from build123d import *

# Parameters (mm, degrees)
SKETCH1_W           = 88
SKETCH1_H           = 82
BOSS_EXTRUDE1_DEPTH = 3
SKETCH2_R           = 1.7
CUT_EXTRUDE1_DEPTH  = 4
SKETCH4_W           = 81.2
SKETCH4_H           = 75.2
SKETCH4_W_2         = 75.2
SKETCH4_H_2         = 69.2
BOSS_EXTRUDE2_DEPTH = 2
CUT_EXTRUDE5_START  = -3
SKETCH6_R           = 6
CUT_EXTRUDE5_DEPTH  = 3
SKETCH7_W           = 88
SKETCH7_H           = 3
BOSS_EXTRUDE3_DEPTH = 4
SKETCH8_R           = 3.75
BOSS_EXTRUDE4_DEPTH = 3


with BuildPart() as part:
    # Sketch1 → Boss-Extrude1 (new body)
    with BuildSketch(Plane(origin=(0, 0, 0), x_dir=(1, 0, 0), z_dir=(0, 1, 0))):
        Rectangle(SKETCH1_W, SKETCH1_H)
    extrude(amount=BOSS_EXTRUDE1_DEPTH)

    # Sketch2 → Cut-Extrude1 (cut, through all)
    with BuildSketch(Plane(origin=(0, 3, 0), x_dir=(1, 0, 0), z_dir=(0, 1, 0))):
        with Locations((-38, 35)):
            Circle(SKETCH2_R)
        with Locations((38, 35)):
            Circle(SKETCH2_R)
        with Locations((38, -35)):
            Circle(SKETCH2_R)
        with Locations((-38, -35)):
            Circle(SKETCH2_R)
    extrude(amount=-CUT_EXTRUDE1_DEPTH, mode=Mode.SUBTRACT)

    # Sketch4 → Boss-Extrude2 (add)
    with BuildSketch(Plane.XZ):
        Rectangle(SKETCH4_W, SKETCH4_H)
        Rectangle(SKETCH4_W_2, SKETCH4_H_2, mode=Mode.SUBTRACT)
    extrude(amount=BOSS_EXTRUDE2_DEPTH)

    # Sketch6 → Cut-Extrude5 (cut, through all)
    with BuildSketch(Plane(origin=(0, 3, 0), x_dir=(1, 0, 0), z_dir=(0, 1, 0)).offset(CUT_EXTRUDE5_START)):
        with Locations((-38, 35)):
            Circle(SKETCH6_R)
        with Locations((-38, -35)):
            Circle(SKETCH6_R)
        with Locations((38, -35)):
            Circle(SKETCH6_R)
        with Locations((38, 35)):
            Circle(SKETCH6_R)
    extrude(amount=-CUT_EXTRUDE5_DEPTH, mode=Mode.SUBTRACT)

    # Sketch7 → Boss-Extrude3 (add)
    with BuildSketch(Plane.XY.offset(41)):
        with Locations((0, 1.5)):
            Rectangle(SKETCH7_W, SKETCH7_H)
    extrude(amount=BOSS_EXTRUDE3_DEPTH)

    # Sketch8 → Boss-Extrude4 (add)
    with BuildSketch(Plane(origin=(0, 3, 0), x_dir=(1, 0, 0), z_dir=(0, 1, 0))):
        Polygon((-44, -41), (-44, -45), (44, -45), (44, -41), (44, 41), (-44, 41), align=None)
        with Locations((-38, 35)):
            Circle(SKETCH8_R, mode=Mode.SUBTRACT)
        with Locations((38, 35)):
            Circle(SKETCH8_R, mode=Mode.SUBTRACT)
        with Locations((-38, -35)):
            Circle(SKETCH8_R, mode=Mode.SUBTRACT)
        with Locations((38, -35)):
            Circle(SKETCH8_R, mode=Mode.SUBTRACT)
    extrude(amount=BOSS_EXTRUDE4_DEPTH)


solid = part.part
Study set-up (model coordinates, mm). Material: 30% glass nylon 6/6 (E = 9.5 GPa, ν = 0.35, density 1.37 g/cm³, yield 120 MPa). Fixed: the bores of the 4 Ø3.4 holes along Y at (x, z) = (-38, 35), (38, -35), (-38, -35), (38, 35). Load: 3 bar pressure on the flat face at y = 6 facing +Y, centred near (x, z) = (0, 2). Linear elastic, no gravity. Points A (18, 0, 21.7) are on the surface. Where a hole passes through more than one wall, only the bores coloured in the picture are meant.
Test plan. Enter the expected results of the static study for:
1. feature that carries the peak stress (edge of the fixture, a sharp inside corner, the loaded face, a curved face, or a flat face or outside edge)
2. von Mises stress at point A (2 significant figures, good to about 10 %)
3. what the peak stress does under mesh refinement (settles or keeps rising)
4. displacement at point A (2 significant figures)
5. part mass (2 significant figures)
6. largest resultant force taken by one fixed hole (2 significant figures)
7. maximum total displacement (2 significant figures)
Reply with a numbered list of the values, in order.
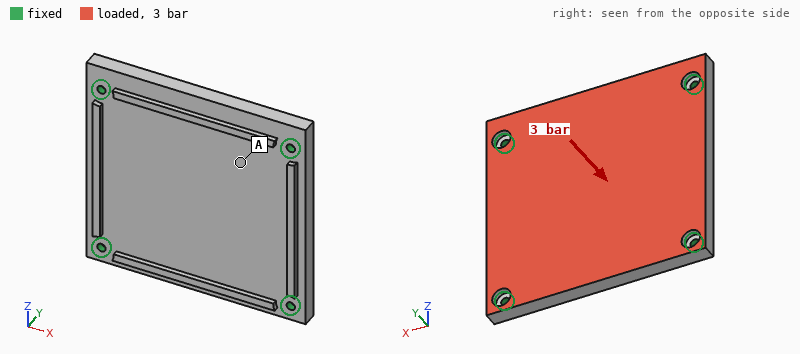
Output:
1. edge of the fixture
2. 10 MPa
3. keeps rising
4. 0.36 mm
5. 63 g
6. 880 N
7. 0.53 mm
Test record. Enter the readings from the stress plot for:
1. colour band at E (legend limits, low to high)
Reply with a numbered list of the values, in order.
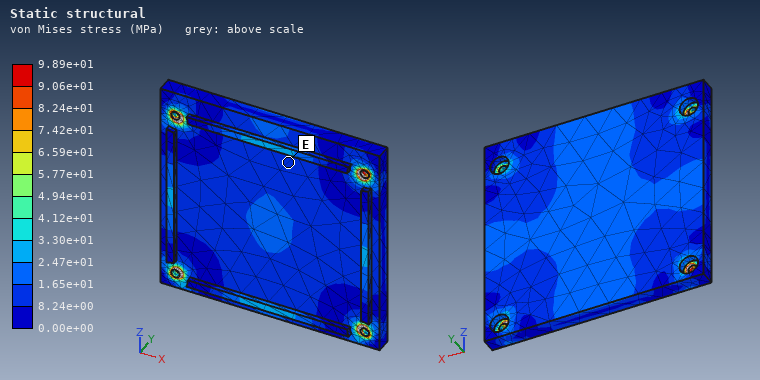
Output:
1. 8.24e+00 to 1.65e+01 MPa
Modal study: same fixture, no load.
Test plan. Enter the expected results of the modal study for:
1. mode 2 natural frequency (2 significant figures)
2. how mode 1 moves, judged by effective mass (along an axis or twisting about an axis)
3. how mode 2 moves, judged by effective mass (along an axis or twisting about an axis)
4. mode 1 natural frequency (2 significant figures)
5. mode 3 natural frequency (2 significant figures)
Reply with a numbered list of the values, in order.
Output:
1. 2500 Hz
2. along Y
3. twisting about X
4. 1600 Hz
5. 2800 Hz
